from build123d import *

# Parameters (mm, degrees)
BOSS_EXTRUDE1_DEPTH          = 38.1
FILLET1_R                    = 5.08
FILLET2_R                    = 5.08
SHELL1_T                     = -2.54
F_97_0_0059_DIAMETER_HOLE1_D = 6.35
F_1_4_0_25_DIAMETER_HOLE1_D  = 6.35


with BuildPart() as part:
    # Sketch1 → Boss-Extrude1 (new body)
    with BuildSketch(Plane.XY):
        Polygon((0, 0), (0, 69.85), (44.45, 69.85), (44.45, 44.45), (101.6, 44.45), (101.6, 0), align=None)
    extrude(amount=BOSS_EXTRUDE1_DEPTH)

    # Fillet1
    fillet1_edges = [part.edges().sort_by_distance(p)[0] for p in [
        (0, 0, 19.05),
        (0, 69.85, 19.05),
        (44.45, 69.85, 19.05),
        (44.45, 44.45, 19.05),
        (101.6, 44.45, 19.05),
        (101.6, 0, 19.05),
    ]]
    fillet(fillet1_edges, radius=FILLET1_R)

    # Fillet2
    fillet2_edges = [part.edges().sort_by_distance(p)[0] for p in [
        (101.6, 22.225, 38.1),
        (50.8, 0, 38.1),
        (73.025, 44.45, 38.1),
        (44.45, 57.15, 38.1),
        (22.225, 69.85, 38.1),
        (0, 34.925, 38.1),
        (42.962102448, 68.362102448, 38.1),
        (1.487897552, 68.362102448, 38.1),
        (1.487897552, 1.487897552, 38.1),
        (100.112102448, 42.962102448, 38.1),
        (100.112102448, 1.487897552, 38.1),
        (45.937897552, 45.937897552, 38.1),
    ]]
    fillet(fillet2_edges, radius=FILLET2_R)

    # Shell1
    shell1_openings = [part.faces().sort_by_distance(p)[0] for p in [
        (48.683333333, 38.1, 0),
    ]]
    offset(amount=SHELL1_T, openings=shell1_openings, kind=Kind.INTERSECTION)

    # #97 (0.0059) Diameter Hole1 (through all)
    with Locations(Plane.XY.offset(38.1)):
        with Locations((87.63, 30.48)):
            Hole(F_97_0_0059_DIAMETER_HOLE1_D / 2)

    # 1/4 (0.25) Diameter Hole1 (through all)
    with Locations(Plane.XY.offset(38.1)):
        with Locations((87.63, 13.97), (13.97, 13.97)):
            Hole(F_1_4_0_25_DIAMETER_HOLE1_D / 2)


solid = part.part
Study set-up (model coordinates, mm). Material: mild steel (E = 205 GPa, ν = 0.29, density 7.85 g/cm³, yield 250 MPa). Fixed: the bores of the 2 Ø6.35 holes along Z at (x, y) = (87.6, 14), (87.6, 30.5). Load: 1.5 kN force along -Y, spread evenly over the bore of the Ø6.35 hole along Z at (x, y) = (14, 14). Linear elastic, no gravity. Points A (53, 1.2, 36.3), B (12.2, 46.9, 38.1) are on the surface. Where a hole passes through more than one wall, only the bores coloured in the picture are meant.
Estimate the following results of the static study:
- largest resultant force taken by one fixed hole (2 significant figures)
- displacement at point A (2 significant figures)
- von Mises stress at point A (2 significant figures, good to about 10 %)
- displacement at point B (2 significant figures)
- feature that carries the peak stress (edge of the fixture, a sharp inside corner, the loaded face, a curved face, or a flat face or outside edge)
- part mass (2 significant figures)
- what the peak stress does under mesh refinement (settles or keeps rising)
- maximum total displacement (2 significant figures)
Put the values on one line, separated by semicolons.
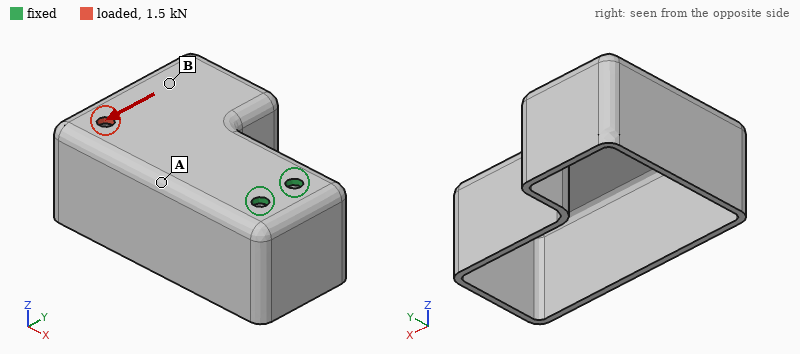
5.1 kN; 0.037 mm; 38 MPa; 0.084 mm; edge of the fixture; 330 g; keeps rising; 0.12 mm
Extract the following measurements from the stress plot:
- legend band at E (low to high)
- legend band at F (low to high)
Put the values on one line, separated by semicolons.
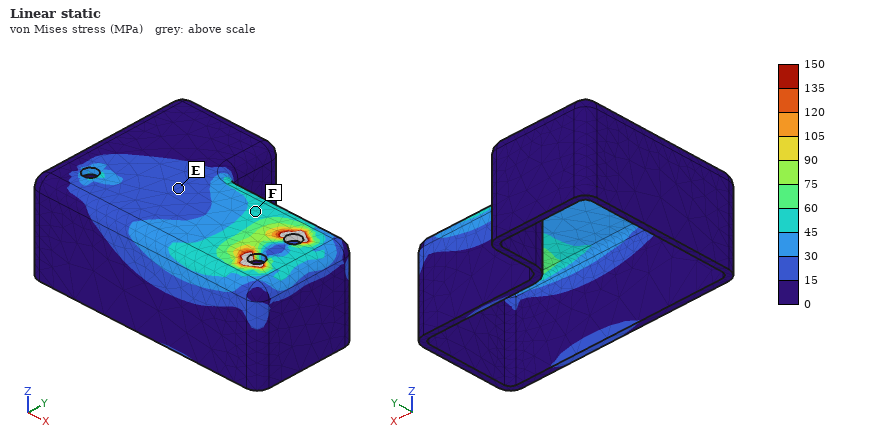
15 to 30 MPa; 45 to 60 MPa
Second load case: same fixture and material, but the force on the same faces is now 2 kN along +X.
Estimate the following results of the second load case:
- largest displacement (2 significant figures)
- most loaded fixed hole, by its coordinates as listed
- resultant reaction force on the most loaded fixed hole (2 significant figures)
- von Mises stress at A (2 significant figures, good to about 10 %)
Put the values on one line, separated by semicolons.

22 µm; (87.6, 14); 1.8 kN; 23 MPa
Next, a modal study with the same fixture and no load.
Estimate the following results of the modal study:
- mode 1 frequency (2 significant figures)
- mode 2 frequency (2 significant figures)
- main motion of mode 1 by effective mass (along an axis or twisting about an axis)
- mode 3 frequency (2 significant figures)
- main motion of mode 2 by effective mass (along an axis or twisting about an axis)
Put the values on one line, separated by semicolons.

330 Hz; 540 Hz; along Z; 1500 Hz; along Y
